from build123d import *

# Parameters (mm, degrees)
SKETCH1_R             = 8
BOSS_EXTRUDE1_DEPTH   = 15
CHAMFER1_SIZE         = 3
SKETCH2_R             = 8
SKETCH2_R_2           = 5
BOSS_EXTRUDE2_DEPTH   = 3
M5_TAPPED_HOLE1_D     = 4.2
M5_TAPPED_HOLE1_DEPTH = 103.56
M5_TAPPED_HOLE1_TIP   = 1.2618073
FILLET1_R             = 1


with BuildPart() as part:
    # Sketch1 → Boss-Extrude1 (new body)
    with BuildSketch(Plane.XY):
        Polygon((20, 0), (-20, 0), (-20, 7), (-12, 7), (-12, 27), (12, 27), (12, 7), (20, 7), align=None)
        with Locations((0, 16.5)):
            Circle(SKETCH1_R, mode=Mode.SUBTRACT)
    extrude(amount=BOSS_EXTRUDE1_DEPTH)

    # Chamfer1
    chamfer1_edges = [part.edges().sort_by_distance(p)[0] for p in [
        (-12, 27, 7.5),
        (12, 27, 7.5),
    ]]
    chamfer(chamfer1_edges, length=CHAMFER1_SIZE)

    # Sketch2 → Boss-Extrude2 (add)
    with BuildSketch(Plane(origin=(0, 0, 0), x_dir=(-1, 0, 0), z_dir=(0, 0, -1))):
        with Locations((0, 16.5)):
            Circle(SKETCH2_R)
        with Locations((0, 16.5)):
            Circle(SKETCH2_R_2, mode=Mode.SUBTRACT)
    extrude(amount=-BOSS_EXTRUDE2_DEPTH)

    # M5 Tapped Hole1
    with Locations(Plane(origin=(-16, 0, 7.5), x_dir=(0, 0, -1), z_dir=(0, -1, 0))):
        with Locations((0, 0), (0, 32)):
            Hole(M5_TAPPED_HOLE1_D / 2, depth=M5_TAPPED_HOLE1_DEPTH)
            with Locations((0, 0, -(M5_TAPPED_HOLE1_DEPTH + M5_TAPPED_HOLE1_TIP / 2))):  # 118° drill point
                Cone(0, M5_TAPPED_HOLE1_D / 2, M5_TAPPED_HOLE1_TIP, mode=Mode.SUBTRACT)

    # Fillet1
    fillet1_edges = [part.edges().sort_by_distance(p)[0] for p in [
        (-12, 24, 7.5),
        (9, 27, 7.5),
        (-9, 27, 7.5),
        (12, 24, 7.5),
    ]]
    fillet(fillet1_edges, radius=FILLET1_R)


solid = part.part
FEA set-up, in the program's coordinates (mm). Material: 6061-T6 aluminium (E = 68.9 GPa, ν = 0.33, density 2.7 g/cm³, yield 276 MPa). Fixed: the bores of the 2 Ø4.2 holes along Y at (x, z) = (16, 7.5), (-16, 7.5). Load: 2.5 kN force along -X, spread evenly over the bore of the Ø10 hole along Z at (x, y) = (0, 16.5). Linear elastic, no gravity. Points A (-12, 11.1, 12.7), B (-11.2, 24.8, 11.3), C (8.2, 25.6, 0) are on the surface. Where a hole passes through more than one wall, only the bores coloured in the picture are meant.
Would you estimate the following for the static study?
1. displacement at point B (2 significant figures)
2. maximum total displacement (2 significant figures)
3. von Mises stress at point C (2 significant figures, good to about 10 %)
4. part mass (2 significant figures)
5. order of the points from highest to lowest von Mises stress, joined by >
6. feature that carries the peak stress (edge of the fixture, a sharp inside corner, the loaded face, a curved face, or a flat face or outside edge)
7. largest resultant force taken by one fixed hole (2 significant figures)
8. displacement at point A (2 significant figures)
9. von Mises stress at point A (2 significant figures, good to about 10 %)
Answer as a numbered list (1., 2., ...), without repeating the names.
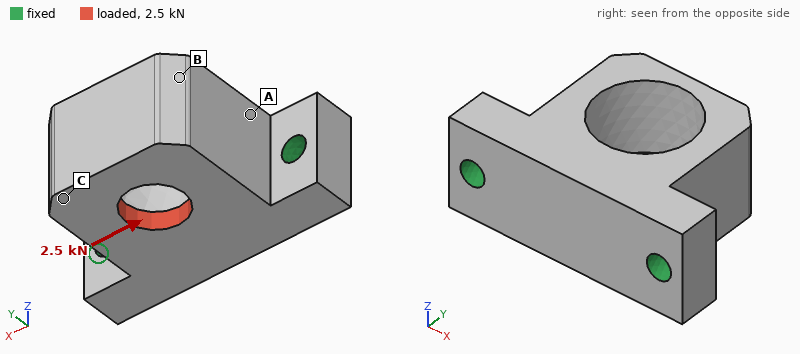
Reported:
1. 23 µm
2. 30 µm
3. 21 MPa
4. 23 g
5. A > C > B
6. the loaded face
7. 1.8 kN
8. 7.1 µm
9. 32 MPa
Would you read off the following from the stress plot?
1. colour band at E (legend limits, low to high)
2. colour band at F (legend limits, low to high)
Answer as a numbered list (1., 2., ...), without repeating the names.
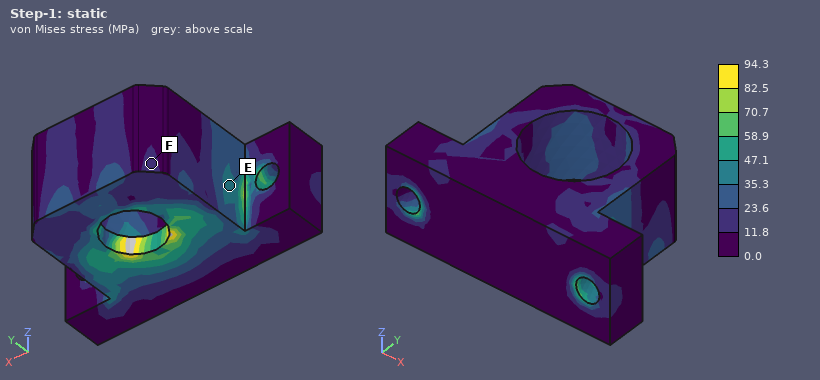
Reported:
1. 35.3 to 47.1 MPa
2. 11.8 to 23.6 MPa
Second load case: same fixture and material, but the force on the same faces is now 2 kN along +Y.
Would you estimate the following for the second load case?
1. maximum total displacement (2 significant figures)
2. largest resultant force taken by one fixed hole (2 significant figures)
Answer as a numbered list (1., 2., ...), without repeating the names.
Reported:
1. 36 µm
2. 1.1 kN
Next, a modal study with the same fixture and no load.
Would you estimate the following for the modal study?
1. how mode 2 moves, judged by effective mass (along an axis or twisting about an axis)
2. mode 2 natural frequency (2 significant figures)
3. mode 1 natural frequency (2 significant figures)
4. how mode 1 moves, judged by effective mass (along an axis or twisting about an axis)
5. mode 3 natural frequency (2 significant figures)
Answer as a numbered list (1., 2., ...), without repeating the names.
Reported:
1. along X
2. 14 kHz
3. 8600 Hz
4. along Z
5. 22 kHz
